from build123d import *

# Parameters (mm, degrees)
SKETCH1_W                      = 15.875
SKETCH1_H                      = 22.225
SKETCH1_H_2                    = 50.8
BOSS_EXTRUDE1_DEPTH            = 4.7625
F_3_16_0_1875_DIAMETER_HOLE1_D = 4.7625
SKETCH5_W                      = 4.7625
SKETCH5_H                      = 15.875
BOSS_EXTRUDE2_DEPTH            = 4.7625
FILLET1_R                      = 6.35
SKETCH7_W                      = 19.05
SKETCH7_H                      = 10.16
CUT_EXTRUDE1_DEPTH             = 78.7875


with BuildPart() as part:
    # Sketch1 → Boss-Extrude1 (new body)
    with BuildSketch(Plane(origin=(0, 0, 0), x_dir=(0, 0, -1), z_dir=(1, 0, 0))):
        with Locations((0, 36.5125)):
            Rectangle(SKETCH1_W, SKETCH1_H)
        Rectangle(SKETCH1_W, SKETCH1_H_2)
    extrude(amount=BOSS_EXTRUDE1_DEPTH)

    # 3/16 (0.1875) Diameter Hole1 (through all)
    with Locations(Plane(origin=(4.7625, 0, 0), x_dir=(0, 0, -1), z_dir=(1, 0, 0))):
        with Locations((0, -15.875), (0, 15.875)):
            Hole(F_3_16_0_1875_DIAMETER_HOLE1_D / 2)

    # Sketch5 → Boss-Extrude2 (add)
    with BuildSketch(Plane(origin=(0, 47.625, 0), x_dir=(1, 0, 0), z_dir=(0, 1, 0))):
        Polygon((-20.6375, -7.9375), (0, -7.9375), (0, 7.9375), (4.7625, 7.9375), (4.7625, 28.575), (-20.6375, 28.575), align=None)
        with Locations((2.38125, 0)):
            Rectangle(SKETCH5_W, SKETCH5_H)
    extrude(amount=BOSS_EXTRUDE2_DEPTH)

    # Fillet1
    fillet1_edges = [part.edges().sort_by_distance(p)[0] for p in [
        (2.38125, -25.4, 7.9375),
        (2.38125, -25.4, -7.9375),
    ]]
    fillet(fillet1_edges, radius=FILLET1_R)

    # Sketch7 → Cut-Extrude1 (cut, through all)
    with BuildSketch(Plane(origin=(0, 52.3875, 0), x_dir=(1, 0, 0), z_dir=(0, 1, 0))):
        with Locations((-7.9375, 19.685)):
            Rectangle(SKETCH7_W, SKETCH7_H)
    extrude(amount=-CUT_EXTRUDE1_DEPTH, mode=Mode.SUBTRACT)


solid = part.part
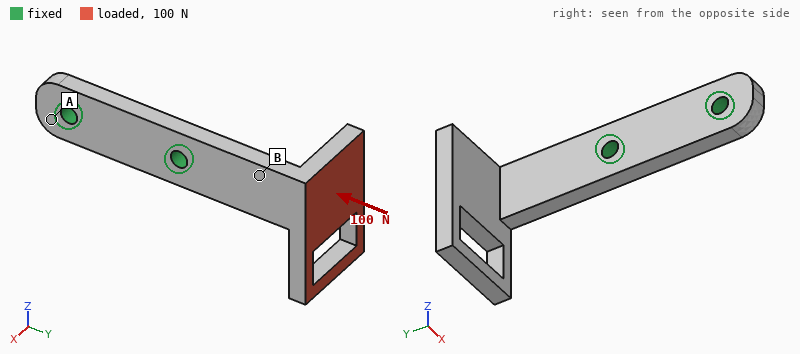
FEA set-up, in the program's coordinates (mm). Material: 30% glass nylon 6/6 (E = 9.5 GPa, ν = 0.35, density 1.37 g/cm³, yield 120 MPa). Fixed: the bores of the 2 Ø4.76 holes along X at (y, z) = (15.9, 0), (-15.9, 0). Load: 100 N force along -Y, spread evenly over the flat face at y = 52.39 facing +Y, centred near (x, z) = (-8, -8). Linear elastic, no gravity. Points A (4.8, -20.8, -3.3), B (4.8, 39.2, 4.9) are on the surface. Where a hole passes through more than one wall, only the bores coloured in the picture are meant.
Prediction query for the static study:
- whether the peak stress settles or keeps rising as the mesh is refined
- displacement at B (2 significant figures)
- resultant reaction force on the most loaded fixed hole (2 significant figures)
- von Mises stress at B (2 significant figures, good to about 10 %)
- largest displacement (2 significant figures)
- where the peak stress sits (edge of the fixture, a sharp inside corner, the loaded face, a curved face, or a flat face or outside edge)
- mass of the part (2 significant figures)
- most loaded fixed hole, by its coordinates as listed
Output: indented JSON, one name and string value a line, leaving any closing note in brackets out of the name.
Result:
{
  "whether the peak stress settles or keeps rising as the mesh is refined": "keeps rising",
  "displacement at B": "0.19 mm",
  "resultant reaction force on the most loaded fixed hole": "94 N",
  "von Mises stress at B": "18 MPa",
  "largest displacement": "0.95 mm",
  "where the peak stress sits": "edge of the fixture",
  "mass of the part": "12 g",
  "most loaded fixed hole, by its coordinates as listed": "(15.9, 0)"
}
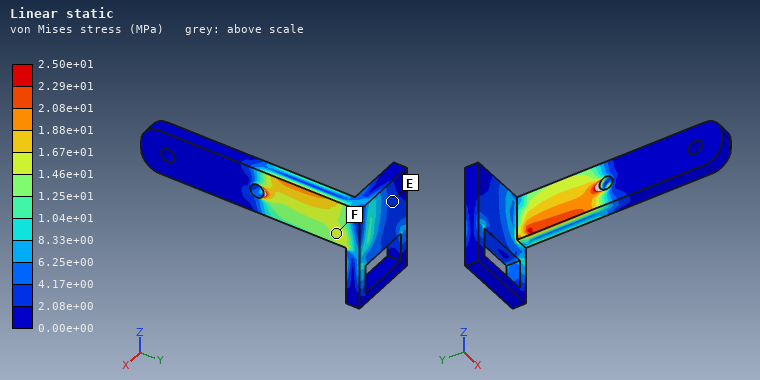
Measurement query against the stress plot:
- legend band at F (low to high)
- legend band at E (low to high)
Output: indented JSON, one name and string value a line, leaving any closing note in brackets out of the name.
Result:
{
  "legend band at F": "1.46e+01 to 1.67e+01 MPa",
  "legend band at E": "2.08e+00 to 4.17e+00 MPa"
}
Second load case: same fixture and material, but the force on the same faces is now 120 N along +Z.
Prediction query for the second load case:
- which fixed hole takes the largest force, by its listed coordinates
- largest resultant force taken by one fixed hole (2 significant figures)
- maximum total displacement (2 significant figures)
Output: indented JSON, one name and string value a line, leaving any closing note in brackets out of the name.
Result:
{
  "which fixed hole takes the largest force, by its listed coordinates": "(15.9, 0)",
  "largest resultant force taken by one fixed hole": "190 N",
  "maximum total displacement": "0.99 mm"
}
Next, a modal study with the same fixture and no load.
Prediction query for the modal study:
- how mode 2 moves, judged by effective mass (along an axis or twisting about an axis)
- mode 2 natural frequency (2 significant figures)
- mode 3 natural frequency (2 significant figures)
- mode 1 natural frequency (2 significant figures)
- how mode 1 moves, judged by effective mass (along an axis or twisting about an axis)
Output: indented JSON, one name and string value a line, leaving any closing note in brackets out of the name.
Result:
{
  "how mode 2 moves, judged by effective mass": "along Z",
  "mode 2 natural frequency": "950 Hz",
  "mode 3 natural frequency": "1800 Hz",
  "mode 1 natural frequency": "600 Hz",
  "how mode 1 moves, judged by effective mass": "along X"
}
